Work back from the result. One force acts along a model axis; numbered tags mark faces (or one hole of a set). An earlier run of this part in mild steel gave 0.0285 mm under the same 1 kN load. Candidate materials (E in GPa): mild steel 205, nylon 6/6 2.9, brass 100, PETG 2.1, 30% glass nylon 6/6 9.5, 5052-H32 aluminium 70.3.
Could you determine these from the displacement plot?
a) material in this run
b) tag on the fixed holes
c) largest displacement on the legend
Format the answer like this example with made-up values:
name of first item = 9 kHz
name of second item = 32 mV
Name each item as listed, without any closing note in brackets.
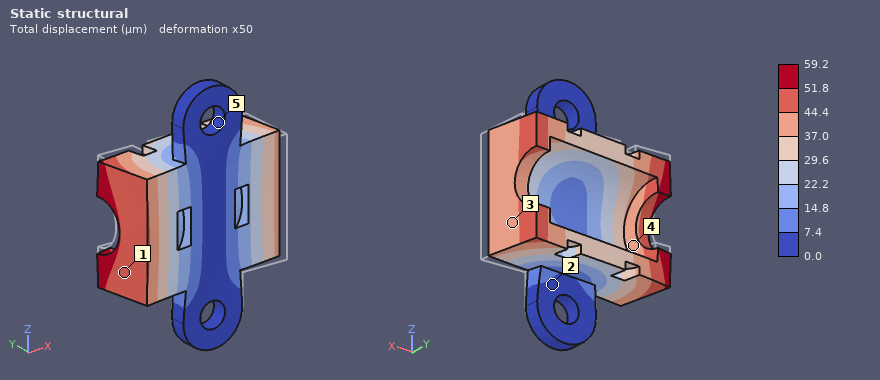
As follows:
material in this run = brass
tag on the fixed holes = 5
largest displacement on the legend = 59.2 µm
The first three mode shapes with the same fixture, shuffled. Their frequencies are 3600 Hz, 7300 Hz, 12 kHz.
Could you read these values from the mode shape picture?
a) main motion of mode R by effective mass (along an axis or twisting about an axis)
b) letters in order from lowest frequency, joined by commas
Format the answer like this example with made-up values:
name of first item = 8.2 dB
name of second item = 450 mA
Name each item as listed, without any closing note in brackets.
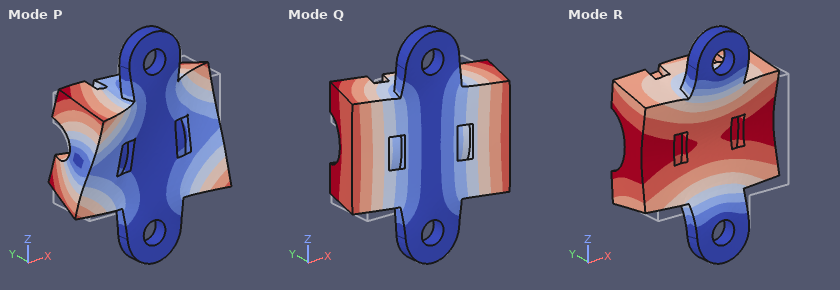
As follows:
main motion of mode R by effective mass = along Y
letters in order from lowest frequency, joined by commas = Q, R, P
